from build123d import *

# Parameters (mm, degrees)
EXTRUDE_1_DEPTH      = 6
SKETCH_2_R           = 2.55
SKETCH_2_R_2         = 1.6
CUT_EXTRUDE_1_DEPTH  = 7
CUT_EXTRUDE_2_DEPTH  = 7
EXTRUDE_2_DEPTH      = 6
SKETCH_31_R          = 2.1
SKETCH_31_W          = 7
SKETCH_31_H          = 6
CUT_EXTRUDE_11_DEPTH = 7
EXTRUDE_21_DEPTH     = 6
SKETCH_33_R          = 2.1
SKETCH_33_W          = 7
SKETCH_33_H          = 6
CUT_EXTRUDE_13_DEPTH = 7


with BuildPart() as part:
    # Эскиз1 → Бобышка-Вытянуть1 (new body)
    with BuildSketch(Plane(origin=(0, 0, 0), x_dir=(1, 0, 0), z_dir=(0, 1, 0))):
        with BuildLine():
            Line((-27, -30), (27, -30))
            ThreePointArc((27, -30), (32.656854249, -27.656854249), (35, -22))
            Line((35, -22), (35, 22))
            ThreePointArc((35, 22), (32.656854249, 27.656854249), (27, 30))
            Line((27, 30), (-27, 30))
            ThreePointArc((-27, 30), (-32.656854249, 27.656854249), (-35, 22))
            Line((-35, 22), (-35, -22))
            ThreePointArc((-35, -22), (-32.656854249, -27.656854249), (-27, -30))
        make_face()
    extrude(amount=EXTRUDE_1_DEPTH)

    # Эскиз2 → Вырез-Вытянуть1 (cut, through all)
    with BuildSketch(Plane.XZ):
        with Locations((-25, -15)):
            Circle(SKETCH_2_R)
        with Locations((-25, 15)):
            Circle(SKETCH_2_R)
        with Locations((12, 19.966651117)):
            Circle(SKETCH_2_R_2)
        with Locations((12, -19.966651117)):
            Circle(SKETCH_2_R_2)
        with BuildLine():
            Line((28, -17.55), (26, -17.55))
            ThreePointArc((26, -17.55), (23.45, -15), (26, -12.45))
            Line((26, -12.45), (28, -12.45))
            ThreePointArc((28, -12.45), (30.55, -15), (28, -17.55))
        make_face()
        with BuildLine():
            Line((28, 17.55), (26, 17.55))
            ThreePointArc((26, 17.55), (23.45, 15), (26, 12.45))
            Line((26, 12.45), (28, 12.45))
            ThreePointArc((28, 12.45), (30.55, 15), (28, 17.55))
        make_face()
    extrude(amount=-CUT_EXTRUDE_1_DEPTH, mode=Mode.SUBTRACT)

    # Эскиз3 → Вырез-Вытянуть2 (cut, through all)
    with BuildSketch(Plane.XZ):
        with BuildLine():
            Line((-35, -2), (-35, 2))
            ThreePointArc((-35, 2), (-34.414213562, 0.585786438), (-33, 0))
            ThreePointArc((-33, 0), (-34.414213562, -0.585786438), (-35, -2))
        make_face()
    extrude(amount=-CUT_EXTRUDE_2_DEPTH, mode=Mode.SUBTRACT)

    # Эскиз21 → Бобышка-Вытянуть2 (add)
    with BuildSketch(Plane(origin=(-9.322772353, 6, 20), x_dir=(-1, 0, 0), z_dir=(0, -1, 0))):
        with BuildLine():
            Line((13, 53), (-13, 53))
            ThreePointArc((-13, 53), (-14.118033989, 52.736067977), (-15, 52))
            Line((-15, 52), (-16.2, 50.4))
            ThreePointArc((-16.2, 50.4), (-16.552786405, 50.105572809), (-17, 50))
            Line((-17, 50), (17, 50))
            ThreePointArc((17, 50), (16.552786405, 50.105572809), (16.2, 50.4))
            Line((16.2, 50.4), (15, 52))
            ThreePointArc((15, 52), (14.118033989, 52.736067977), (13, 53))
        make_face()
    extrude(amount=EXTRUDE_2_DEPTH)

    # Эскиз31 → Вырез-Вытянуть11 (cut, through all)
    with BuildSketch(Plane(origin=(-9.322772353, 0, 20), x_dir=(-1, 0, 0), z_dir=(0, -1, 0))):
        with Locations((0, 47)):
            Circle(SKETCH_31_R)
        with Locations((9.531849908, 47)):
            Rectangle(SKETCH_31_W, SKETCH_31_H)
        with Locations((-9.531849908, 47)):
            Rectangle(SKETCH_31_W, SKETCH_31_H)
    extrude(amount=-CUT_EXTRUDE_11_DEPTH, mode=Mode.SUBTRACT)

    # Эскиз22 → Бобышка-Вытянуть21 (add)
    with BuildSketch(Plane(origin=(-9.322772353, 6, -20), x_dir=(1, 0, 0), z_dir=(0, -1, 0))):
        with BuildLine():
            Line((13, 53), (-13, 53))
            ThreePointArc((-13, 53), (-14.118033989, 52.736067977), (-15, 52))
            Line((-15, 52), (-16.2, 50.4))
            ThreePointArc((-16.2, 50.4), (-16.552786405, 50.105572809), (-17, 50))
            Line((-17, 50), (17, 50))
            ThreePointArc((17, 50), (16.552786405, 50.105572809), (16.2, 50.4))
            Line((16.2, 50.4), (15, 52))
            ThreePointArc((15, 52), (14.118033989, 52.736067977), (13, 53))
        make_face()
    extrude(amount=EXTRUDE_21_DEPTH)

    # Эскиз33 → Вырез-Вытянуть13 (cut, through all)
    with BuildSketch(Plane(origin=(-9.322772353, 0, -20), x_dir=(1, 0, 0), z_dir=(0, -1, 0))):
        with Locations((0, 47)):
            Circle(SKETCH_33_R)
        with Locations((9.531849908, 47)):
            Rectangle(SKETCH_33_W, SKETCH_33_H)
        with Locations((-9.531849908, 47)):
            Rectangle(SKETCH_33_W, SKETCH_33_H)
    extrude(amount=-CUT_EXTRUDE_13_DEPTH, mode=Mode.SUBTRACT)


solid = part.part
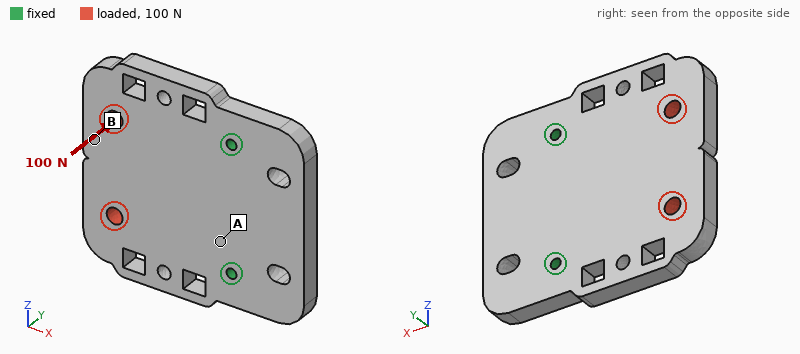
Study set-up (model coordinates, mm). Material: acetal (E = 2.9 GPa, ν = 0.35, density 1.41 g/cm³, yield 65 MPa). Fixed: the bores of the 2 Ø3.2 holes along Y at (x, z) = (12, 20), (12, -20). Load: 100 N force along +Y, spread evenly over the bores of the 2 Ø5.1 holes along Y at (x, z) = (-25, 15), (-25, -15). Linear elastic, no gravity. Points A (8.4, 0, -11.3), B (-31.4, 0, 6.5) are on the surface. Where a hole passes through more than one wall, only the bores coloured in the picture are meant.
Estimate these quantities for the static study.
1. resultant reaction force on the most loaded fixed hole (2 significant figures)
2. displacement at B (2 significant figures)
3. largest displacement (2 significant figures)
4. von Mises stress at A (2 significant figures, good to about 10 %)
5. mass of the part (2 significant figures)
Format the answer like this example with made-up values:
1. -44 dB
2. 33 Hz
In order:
1. 50 N
2. 0.97 mm
3. 1.1 mm
4. 7.0 MPa
5. 34 g
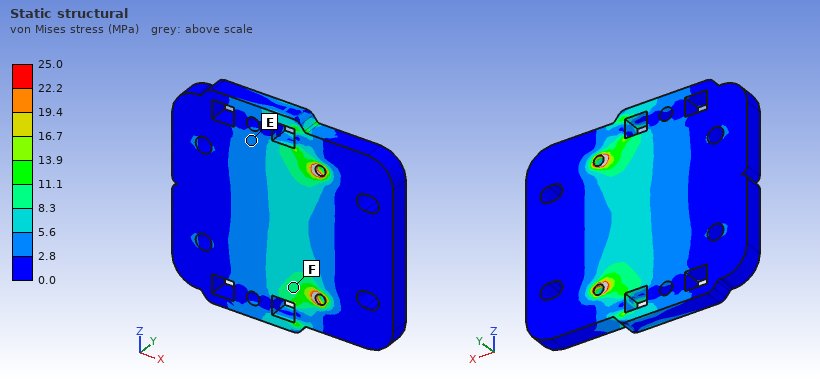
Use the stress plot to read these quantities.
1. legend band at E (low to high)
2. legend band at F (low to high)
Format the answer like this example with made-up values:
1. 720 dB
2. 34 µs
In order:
1. 2.8 to 5.6 MPa
2. 8.3 to 11.1 MPa
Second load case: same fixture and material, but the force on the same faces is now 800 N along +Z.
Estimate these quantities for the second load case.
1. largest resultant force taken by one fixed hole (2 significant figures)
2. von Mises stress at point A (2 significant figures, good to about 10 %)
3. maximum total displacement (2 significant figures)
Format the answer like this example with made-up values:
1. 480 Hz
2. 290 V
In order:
1. 820 N
2. 5.1 MPa
3. 0.22 mm
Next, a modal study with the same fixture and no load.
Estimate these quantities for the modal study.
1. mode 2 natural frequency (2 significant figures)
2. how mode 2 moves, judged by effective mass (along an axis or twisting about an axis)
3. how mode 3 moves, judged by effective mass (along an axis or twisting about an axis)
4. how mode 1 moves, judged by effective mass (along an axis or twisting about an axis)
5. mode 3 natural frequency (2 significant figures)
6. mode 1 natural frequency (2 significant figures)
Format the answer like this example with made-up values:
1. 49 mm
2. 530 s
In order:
1. 1200 Hz
2. twisting about X
3. along Y
4. along Y
5. 2000 Hz
6. 540 Hz
